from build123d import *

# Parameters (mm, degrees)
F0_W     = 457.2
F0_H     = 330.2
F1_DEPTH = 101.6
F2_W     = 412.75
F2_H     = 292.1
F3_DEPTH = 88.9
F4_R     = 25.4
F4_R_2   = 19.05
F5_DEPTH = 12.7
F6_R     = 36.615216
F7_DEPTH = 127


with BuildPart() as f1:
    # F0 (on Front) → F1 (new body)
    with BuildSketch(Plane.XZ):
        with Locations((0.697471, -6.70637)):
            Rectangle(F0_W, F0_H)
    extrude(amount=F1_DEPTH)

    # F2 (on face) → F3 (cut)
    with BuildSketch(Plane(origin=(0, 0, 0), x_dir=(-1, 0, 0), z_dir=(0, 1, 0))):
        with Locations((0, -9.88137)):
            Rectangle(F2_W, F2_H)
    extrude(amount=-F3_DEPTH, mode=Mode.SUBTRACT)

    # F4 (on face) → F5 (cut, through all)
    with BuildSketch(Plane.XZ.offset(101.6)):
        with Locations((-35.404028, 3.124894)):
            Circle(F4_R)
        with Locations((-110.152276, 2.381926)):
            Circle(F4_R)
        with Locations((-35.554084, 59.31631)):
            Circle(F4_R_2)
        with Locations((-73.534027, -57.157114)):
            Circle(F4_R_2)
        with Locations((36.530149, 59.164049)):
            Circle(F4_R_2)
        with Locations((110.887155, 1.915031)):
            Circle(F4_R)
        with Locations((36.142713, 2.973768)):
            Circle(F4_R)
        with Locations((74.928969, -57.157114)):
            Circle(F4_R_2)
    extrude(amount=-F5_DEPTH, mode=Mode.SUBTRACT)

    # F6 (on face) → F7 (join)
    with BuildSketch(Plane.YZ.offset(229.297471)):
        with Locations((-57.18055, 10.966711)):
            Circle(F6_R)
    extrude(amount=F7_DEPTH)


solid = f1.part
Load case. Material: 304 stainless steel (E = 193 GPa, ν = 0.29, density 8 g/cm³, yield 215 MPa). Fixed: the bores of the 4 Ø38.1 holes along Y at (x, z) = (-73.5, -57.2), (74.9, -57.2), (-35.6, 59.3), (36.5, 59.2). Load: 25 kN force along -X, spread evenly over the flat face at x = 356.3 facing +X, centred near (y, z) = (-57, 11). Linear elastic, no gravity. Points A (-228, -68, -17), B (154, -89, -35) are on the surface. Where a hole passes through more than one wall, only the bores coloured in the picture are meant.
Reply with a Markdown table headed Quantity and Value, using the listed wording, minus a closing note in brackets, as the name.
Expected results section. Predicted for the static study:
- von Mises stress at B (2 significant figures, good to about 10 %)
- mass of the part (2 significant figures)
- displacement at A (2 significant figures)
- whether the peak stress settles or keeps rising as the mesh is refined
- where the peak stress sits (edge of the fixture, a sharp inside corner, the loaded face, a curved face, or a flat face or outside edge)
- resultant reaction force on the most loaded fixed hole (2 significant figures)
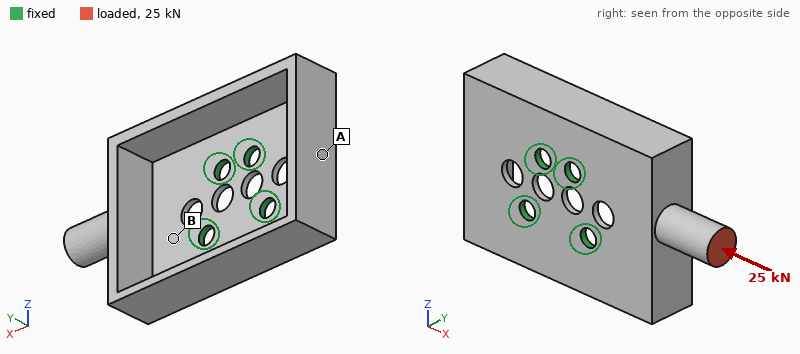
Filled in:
| Quantity | Value |
|---|---|
| von Mises stress at B | 24 MPa |
| mass of the part | 40 kg |
| displacement at A | 0.10 mm |
| whether the peak stress settles or keeps rising as the mesh is refined | keeps rising |
| where the peak stress sits | edge of the fixture |
| resultant reaction force on the most loaded fixed hole | 11 kN |
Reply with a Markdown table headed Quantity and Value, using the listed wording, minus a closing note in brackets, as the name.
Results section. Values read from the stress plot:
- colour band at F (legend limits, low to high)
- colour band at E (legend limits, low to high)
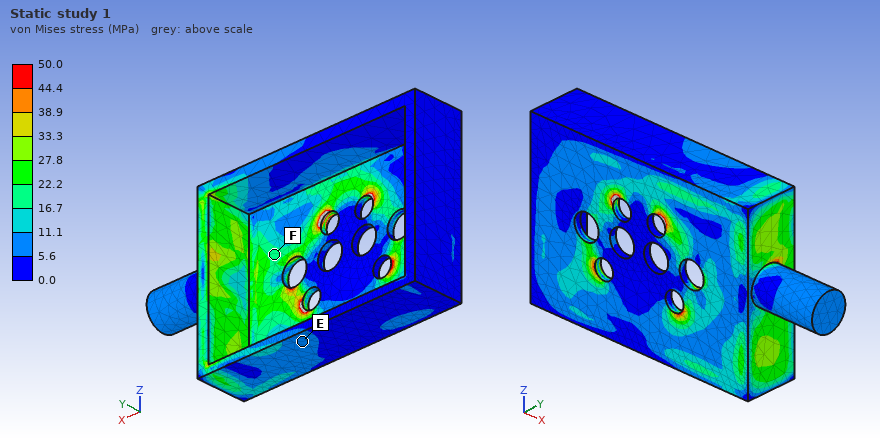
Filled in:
| Quantity | Value |
|---|---|
| colour band at F | 16.7 to 22.2 MPa |
| colour band at E | 5.6 to 11.1 MPa |
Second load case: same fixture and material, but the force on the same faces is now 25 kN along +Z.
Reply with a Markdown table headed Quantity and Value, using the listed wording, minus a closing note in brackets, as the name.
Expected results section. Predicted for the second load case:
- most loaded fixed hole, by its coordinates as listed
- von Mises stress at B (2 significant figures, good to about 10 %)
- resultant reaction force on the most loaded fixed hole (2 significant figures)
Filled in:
| Quantity | Value |
|---|---|
| most loaded fixed hole, by its coordinates as listed | (74.9, -57.2) |
| von Mises stress at B | 36 MPa |
| resultant reaction force on the most loaded fixed hole | 37 kN |
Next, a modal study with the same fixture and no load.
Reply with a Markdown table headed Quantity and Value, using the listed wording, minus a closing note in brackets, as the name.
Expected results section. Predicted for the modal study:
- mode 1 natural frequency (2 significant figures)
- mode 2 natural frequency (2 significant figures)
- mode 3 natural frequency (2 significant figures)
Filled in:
| Quantity | Value |
|---|---|
| mode 1 natural frequency | 200 Hz |
| mode 2 natural frequency | 340 Hz |
| mode 3 natural frequency | 350 Hz |
